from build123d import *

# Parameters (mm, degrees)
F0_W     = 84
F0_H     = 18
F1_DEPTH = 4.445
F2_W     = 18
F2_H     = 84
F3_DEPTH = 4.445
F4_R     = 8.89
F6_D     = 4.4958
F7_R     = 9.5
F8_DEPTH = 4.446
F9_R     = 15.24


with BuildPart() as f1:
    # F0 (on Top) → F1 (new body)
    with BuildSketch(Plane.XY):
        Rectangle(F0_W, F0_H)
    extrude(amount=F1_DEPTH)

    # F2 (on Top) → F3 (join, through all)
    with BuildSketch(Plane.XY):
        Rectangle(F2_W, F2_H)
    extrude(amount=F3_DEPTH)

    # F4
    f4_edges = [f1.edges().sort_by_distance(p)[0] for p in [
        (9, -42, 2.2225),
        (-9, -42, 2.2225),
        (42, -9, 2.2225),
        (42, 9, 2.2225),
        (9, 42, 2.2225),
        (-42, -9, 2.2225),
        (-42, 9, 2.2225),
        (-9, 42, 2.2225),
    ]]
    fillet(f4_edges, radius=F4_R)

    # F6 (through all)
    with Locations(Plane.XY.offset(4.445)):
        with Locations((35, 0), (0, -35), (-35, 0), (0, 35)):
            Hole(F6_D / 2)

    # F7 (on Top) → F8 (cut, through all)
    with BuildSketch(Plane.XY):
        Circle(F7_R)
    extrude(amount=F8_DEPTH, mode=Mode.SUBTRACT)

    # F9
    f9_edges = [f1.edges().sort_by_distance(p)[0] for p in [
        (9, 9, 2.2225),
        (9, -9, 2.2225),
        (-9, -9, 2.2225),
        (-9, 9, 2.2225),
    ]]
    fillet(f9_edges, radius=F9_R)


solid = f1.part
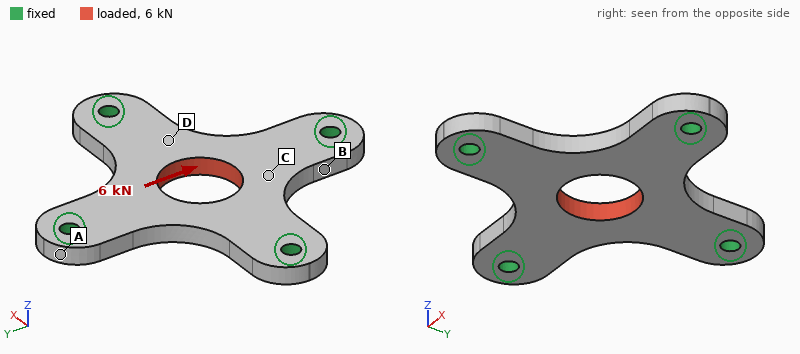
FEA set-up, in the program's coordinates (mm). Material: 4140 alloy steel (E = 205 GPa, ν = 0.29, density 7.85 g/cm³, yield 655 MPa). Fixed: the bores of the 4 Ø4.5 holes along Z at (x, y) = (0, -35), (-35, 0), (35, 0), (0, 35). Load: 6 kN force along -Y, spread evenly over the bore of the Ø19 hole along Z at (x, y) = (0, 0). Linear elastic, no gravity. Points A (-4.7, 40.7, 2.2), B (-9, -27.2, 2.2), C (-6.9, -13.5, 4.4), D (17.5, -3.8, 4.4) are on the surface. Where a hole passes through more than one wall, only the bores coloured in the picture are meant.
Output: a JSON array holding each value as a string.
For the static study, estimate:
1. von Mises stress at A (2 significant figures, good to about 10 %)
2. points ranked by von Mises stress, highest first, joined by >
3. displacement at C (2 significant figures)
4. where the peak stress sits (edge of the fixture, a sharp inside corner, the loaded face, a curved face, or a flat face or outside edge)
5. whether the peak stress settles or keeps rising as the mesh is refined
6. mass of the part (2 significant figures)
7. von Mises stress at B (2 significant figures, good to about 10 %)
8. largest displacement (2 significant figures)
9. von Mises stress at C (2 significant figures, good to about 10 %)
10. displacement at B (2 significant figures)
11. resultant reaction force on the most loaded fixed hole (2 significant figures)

["15 MPa", "C > B > A > D", "4.0 µm", "edge of the fixture", "keeps rising", "84 g", "24 MPa", "5.9 µm", "37 MPa", "2.0 µm", "2.6 kN"]
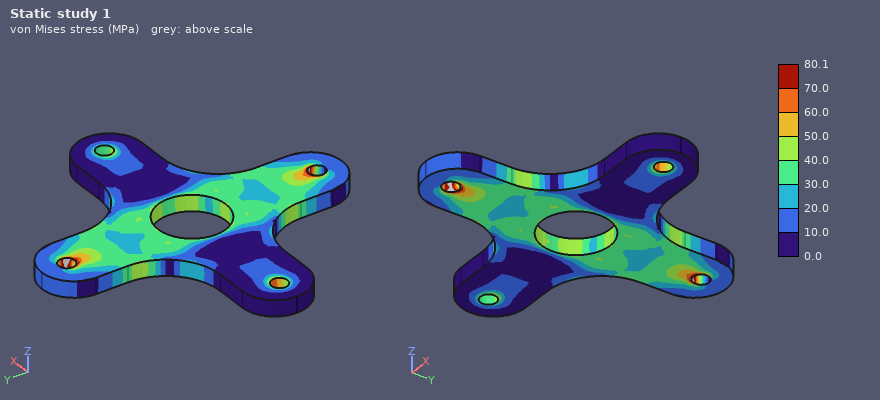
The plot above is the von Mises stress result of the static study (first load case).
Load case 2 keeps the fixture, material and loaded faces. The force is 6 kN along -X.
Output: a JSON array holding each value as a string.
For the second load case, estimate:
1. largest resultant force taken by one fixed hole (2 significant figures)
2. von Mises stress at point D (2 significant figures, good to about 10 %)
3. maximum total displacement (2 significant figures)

["2.6 kN", "30 MPa", "5.9 µm"]
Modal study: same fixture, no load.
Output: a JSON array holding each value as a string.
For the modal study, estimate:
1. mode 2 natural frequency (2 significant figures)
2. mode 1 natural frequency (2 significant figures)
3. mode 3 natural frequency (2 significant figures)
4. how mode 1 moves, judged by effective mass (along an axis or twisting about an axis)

["12 kHz", "6600 Hz", "12 kHz", "along Z"]
